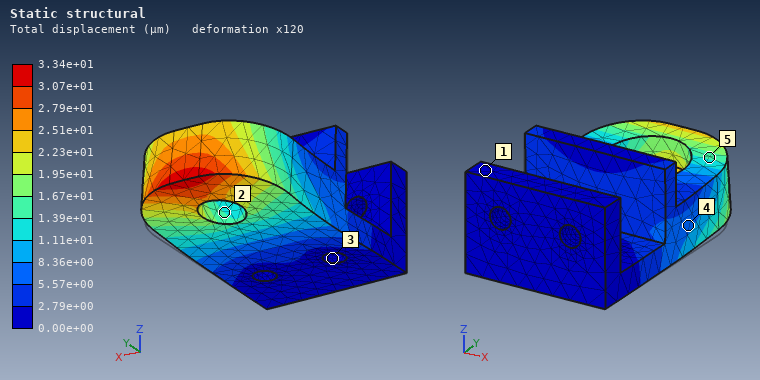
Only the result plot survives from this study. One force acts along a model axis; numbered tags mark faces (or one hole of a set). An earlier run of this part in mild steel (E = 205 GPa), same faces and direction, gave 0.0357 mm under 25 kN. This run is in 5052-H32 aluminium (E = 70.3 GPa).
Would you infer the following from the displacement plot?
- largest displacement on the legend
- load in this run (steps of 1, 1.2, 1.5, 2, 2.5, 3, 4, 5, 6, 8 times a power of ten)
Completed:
3.34e+01 µm
8 kN
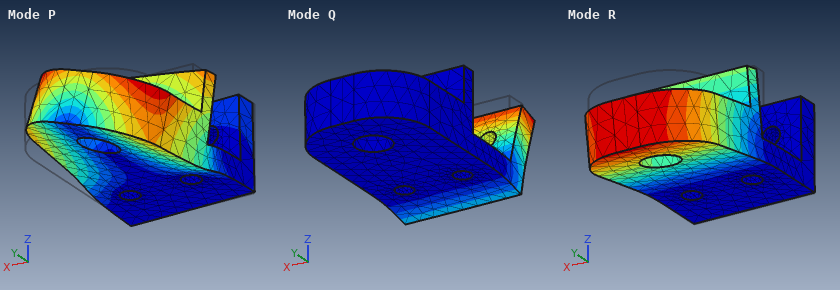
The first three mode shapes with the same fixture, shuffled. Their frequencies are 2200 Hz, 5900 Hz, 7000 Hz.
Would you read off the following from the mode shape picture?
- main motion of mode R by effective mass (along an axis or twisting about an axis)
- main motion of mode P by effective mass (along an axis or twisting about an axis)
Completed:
along Z
along X
